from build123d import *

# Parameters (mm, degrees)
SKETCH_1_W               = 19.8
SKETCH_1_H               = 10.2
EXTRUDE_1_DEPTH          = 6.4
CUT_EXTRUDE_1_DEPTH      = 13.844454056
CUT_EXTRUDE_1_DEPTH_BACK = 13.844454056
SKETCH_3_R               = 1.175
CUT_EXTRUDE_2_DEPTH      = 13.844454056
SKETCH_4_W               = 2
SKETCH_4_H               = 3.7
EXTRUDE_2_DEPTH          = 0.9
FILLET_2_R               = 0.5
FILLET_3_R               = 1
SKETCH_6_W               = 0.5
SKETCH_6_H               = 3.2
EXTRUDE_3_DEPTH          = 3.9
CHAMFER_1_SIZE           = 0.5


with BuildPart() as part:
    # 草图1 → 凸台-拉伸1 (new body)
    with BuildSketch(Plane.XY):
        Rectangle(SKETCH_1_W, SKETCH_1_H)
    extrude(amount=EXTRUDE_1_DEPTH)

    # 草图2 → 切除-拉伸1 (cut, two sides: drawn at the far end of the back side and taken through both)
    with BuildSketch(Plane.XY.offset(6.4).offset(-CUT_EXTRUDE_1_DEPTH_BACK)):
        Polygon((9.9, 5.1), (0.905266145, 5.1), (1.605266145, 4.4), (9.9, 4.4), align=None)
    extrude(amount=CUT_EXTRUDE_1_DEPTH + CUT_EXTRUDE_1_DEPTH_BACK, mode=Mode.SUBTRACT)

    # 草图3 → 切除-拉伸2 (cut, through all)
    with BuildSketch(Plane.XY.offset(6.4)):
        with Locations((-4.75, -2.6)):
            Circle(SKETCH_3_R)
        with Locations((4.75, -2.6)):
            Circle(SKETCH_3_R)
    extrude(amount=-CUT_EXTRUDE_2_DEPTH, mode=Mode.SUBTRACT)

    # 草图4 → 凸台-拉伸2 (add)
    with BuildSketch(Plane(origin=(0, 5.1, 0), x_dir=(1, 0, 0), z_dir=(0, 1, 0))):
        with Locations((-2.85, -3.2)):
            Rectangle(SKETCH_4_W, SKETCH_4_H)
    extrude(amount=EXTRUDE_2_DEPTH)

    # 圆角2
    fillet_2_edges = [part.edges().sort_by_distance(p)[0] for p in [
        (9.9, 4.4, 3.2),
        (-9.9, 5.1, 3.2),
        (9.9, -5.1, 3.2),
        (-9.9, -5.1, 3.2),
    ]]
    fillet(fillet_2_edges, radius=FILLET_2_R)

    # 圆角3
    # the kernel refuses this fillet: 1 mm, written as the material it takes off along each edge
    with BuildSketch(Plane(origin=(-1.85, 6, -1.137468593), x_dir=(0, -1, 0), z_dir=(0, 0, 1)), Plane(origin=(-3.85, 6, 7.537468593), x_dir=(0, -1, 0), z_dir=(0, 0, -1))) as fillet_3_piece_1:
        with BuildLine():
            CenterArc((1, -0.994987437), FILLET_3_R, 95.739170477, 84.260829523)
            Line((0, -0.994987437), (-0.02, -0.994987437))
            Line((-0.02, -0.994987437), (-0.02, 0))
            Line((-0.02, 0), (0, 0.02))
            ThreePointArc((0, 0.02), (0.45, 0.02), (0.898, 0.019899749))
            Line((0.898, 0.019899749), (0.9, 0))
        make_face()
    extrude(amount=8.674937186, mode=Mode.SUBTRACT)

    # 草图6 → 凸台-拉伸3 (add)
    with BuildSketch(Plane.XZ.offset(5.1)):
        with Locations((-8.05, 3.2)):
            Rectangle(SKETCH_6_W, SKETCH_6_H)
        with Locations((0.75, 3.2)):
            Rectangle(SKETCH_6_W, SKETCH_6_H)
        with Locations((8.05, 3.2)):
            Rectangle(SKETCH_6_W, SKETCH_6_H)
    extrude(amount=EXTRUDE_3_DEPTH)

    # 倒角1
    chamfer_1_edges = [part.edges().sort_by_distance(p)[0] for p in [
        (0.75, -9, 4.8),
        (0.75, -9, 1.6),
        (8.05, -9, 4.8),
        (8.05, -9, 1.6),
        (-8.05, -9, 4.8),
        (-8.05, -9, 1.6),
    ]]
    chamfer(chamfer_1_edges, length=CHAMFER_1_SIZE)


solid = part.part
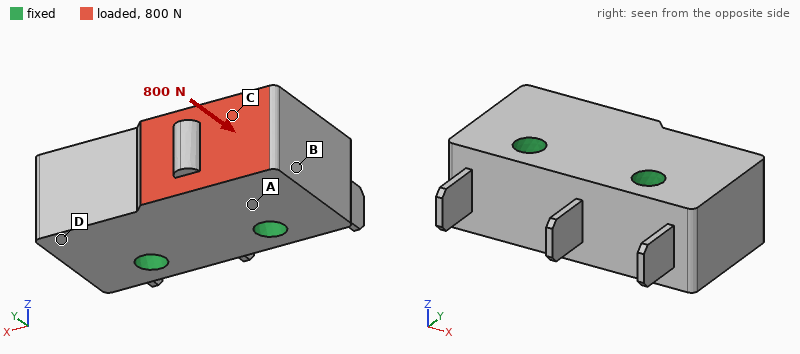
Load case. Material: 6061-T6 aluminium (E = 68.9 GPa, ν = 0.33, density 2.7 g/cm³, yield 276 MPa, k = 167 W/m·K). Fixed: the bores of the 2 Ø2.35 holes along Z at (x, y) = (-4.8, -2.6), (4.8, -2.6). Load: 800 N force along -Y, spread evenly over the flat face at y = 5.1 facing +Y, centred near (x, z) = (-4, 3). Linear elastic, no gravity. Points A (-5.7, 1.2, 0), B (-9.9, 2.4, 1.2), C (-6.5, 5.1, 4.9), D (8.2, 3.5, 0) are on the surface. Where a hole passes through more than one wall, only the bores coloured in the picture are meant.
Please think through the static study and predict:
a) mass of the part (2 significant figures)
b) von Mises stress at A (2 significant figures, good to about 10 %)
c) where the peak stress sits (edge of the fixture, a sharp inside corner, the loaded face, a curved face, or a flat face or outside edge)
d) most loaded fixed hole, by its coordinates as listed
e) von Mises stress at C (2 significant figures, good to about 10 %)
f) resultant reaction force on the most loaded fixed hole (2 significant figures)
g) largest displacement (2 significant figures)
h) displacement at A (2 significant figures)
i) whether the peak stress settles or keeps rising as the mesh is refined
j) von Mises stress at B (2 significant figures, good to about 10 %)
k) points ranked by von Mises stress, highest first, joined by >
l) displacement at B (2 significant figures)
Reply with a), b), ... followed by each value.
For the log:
a) 3.3 g
b) 17 MPa
c) edge of the fixture
d) (-4.8, -2.6)
e) 13 MPa
f) 720 N
g) 2.6 µm
h) 1.1 µm
i) keeps rising
j) 7.2 MPa
k) A > C > B > D
l) 2.2 µm
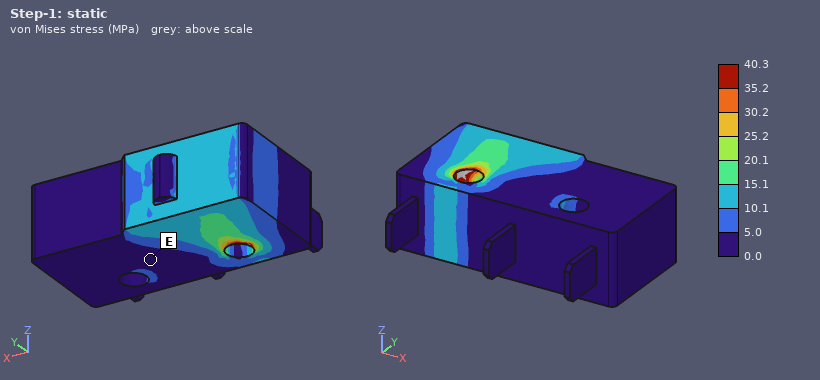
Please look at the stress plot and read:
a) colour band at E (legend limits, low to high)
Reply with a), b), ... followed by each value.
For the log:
a) 0.0 to 5.0 MPa
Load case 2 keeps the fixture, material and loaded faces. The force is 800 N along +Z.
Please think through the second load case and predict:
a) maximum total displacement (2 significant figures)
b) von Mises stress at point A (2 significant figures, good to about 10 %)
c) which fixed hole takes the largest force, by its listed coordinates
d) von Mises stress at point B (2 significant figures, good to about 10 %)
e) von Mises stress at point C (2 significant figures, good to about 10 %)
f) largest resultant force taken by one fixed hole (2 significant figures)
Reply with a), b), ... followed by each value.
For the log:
a) 14 µm
b) 47 MPa
c) (-4.8, -2.6)
d) 18 MPa
e) 30 MPa
f) 640 N
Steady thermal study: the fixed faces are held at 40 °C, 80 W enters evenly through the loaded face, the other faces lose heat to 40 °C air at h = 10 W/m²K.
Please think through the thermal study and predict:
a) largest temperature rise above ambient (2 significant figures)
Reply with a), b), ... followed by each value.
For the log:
a) 52 K
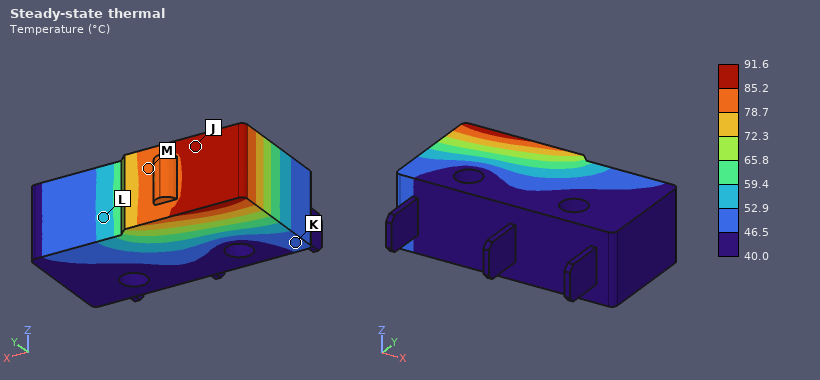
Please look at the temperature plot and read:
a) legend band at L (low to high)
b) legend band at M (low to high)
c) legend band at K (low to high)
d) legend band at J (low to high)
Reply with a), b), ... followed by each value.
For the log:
a) 52.9 to 59.4 °C
b) 78.7 to 85.2 °C
c) 46.5 to 52.9 °C
d) 85.2 to 91.6 °C
